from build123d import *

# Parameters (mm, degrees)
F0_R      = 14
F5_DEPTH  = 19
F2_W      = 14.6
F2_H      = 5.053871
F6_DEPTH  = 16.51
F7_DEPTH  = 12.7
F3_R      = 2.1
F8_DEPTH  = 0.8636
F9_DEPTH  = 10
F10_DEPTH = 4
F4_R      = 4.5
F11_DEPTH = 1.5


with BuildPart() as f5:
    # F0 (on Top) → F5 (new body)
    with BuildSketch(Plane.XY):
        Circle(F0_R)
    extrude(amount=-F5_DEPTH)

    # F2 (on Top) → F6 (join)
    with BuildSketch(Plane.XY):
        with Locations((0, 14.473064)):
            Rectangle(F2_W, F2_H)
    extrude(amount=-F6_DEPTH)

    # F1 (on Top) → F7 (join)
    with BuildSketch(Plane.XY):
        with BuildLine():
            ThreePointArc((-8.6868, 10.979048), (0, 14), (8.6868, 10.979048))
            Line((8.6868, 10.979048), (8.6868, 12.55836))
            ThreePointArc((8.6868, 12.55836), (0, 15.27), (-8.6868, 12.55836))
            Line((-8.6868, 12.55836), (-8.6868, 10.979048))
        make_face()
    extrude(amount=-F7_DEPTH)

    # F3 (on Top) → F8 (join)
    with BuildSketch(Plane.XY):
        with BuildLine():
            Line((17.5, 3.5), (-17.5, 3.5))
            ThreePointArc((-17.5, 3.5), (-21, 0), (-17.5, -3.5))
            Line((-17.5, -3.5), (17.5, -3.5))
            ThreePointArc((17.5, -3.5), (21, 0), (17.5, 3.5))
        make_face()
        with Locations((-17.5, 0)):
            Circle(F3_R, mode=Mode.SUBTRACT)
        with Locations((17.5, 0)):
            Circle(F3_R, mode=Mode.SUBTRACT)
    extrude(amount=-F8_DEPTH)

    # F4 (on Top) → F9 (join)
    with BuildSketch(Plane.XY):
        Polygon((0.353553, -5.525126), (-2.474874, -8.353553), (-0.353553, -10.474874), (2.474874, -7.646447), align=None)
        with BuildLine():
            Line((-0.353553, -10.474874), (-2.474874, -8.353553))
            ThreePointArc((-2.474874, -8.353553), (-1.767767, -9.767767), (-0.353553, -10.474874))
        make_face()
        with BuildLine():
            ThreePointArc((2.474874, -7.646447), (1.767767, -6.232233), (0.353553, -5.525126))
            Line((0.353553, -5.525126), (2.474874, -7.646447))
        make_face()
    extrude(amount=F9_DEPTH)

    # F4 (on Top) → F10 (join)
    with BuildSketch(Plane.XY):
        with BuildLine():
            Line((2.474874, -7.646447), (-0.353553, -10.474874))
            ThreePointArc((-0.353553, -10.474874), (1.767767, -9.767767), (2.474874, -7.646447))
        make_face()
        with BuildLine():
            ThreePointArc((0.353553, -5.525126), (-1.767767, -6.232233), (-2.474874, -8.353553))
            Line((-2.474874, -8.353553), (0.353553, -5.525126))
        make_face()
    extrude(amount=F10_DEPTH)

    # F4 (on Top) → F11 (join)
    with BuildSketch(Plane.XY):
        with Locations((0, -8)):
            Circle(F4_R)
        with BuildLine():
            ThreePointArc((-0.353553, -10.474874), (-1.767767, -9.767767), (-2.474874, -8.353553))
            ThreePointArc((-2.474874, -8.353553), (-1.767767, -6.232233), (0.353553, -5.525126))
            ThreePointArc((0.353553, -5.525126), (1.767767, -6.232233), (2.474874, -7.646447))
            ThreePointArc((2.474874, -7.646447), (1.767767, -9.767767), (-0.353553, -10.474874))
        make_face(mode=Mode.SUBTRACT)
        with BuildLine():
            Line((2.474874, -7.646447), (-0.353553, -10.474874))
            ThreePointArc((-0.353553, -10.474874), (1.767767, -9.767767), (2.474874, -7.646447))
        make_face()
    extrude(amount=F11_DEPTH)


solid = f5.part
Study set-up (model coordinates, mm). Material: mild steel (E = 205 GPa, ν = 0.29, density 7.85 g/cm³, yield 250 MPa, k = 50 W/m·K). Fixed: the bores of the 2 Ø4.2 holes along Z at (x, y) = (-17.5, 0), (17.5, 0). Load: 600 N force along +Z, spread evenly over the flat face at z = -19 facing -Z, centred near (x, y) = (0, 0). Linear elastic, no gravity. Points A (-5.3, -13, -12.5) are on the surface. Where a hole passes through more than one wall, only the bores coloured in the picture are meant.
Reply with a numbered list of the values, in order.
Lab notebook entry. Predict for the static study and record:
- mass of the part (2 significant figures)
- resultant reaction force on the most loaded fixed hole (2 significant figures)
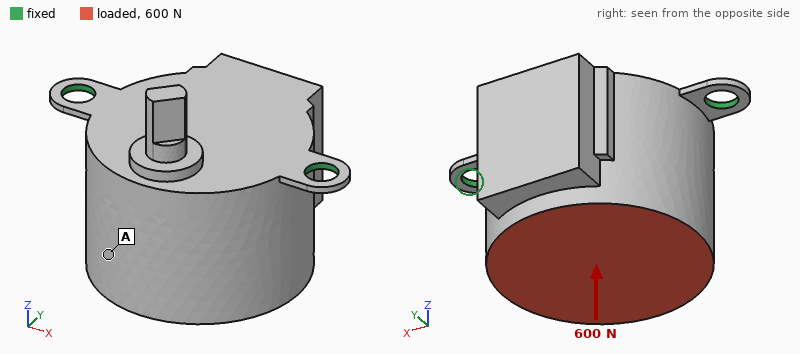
1. 100 g
2. 350 N
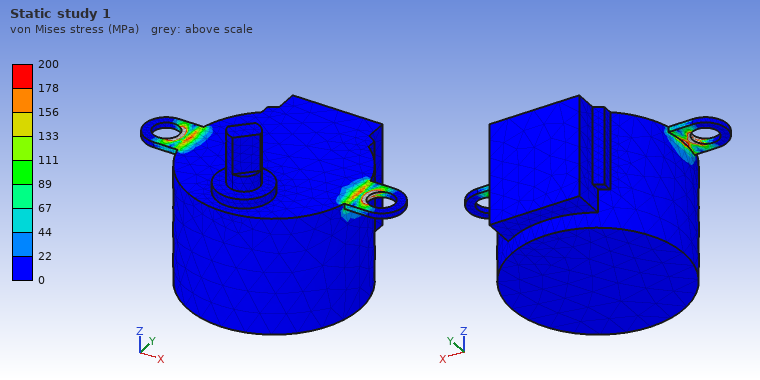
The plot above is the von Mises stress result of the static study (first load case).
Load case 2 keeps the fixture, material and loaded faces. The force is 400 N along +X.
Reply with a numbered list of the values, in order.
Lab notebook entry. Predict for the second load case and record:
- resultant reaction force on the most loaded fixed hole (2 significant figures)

1. 320 N
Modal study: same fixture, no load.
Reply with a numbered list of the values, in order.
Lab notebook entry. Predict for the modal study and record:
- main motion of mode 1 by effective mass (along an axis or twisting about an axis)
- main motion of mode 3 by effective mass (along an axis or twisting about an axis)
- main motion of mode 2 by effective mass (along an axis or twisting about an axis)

1. along Y
2. along X
3. along Z
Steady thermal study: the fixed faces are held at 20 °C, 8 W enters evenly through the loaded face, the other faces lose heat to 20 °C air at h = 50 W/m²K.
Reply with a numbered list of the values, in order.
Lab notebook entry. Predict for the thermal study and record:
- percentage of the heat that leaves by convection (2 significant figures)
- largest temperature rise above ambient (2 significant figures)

1. 44 %
2. 29 K
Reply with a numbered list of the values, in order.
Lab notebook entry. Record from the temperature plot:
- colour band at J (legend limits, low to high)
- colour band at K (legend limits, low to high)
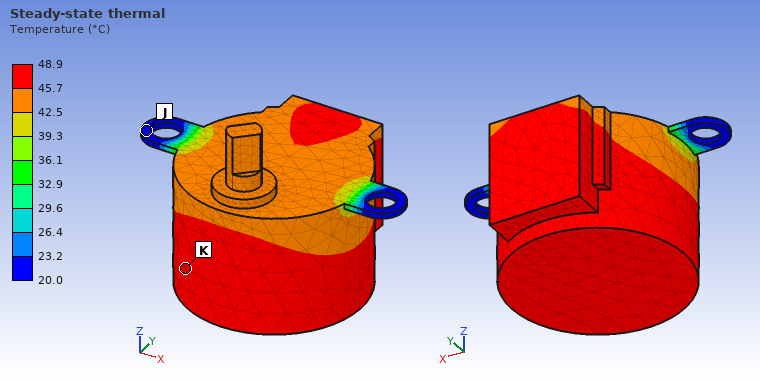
1. 20.0 to 23.2 °C
2. 45.7 to 48.9 °C
